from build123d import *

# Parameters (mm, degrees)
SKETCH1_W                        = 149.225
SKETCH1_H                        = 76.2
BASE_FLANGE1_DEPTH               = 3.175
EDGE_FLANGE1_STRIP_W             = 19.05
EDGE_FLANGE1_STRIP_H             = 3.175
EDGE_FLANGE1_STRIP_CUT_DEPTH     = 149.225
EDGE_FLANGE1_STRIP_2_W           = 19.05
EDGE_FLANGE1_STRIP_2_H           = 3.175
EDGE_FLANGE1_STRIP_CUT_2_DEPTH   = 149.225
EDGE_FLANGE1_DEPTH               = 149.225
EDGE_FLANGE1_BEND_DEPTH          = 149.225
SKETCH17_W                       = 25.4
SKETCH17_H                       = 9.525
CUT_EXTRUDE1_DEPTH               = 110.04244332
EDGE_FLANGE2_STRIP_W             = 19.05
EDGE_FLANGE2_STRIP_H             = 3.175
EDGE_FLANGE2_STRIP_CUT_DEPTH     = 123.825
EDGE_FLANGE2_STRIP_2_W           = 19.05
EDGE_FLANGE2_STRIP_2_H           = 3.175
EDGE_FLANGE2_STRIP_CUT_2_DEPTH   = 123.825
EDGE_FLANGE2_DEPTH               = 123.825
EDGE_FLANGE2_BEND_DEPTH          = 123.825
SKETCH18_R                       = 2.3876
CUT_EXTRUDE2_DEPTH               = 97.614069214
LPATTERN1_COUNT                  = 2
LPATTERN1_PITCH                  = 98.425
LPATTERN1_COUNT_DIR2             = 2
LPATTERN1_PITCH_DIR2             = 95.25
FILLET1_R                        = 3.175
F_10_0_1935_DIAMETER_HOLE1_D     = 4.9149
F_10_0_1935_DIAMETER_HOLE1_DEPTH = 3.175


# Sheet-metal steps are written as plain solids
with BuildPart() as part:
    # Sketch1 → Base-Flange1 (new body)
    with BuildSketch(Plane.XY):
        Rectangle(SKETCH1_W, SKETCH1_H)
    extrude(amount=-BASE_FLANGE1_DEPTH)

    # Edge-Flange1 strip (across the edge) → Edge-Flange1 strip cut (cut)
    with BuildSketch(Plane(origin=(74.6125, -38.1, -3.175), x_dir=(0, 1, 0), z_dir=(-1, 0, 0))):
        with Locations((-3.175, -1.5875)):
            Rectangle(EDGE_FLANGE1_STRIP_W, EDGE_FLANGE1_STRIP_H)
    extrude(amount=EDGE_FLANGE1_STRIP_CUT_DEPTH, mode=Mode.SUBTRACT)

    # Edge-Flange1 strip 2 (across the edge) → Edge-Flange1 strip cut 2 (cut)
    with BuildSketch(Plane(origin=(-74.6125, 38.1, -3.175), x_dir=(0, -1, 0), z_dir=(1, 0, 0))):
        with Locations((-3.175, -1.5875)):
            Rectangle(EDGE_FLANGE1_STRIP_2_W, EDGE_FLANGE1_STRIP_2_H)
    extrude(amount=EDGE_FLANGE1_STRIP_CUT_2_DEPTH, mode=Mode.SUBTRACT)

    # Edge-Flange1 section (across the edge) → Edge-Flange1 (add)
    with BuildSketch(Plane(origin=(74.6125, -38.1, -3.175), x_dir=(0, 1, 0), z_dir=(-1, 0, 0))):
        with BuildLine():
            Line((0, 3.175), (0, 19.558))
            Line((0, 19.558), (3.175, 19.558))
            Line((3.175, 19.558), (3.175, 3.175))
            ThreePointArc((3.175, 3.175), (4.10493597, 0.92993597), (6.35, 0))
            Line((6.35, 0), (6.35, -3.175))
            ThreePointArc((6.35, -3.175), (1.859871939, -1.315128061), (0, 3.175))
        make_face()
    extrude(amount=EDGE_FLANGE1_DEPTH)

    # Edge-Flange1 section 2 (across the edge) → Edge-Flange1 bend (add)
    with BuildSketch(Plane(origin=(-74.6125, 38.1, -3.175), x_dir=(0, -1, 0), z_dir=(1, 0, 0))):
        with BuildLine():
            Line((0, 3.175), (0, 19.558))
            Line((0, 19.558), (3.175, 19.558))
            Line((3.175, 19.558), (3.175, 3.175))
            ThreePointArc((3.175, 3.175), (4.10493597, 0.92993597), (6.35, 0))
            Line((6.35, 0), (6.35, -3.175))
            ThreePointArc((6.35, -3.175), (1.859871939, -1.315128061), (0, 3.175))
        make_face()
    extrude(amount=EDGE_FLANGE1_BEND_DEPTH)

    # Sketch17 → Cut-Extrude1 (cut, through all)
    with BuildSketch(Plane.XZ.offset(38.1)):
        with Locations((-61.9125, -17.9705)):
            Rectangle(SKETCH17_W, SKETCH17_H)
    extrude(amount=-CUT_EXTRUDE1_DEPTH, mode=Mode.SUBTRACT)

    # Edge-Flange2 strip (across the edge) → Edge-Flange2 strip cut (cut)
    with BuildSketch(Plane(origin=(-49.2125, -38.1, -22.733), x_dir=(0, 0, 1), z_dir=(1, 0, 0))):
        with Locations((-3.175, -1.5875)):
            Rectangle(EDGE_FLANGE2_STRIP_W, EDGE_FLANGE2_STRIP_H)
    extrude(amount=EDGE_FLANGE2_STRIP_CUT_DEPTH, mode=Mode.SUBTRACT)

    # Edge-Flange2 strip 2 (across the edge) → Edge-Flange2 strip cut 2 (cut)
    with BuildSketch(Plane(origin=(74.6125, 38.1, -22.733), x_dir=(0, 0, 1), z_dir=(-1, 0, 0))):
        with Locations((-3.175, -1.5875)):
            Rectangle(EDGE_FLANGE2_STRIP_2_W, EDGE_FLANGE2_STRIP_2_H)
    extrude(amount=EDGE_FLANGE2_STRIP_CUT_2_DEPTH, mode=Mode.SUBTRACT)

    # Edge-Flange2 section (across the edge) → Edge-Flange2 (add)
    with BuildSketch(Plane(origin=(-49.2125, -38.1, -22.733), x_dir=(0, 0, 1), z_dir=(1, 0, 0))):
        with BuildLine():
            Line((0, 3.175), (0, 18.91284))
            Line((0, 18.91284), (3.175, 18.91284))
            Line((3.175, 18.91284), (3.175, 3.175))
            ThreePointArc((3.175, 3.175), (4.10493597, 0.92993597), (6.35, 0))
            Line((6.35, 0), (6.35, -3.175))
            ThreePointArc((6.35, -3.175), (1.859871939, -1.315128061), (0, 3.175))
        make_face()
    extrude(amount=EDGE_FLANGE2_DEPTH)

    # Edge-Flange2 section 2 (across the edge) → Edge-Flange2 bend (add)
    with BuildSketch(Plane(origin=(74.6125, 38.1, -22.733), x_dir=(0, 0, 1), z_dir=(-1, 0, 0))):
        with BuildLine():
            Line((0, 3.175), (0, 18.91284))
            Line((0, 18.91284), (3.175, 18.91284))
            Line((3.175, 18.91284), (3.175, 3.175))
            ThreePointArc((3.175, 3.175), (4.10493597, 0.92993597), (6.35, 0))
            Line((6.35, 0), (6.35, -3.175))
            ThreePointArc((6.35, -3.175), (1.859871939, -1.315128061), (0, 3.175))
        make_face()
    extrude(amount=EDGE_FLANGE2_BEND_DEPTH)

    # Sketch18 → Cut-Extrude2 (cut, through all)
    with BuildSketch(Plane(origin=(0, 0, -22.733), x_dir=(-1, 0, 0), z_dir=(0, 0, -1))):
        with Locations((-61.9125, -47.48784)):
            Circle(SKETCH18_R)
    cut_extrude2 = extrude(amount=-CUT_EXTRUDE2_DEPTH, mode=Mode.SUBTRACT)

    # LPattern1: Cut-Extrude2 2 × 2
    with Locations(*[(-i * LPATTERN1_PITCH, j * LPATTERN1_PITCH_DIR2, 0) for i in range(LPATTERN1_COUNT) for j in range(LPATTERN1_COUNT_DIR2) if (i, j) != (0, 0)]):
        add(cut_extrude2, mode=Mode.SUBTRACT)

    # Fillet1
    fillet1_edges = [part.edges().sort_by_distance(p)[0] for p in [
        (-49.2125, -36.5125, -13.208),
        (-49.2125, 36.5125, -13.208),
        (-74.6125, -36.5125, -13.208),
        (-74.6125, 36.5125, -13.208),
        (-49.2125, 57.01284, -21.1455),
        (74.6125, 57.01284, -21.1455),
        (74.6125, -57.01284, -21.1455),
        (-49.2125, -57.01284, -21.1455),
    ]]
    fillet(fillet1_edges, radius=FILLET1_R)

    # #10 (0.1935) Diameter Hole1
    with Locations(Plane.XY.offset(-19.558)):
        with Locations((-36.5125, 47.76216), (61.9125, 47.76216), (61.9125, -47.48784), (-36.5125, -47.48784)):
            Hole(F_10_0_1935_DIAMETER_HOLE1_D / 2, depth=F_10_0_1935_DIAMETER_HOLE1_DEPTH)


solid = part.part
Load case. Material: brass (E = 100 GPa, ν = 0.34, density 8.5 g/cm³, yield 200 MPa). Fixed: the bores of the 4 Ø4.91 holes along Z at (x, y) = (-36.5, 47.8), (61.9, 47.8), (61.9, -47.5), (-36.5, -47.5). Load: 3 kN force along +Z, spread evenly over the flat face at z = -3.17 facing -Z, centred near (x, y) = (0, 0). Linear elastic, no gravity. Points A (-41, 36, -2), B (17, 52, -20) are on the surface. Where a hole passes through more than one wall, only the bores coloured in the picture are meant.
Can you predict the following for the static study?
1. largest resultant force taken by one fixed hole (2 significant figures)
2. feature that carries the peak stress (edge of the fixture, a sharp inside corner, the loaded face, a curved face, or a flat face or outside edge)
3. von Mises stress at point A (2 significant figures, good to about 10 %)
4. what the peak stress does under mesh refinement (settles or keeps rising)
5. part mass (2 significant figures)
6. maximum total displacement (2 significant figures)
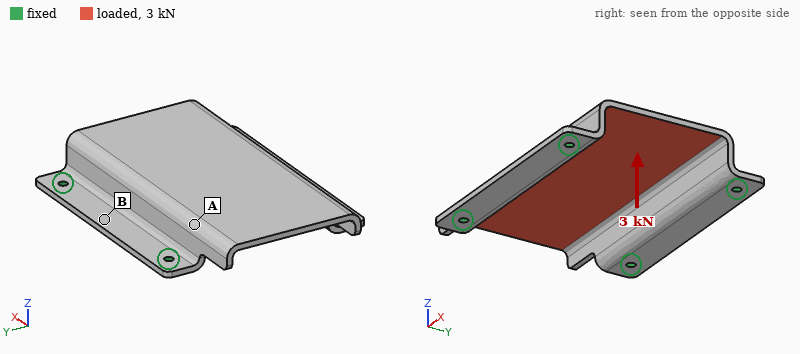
1.3 kN
edge of the fixture
53 MPa
keeps rising
550 g
0.21 mm
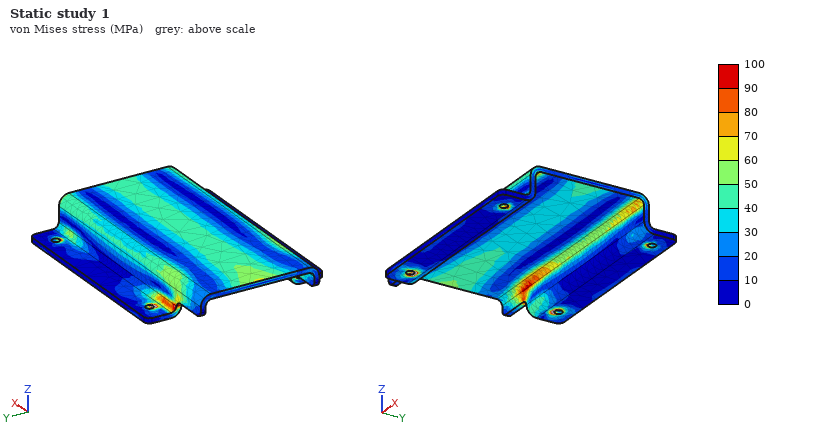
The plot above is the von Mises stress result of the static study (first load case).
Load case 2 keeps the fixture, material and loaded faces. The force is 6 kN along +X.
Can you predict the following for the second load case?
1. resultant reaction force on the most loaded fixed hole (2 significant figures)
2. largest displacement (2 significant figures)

1.7 kN
48 µm
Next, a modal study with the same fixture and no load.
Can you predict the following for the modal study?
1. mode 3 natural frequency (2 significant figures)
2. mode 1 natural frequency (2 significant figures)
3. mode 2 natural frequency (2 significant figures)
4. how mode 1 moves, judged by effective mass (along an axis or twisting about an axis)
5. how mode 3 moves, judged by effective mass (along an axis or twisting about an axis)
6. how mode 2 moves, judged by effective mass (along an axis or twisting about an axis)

1800 Hz
1300 Hz
1500 Hz
along Y
along Z
along Z
